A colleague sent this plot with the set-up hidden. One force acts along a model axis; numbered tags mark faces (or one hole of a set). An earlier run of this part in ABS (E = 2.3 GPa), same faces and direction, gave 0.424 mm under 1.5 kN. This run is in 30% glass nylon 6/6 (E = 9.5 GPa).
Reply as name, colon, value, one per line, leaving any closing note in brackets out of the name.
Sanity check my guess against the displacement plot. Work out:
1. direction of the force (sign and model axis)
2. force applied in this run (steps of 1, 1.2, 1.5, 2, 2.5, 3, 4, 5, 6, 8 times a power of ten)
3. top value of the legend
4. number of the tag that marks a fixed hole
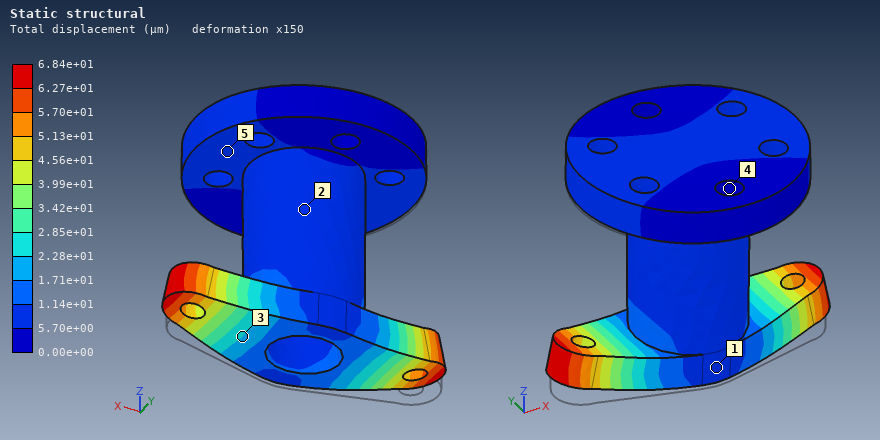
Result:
direction of the force: +Z
force applied in this run: 1 kN
top value of the legend: 6.84e+01 µm
number of the tag that marks a fixed hole: 4
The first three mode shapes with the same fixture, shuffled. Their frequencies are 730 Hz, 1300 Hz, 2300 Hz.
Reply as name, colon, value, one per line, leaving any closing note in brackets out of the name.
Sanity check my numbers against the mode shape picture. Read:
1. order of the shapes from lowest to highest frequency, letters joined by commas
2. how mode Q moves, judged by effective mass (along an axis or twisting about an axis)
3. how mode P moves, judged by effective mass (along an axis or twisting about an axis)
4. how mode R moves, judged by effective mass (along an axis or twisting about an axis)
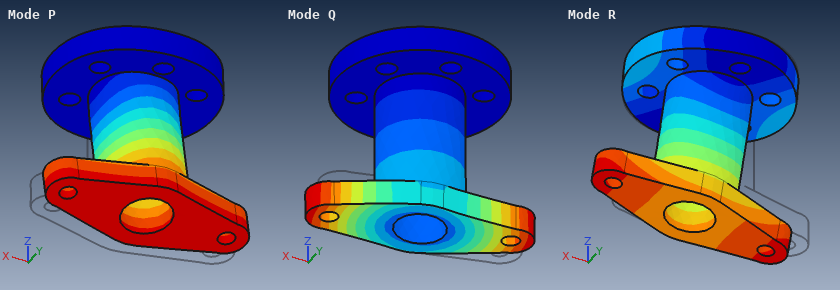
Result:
order of the shapes from lowest to highest frequency, letters joined by commas: R, P, Q
how mode Q moves, judged by effective mass: twisting about Z
how mode P moves, judged by effective mass: along Y
how mode R moves, judged by effective mass: along X
